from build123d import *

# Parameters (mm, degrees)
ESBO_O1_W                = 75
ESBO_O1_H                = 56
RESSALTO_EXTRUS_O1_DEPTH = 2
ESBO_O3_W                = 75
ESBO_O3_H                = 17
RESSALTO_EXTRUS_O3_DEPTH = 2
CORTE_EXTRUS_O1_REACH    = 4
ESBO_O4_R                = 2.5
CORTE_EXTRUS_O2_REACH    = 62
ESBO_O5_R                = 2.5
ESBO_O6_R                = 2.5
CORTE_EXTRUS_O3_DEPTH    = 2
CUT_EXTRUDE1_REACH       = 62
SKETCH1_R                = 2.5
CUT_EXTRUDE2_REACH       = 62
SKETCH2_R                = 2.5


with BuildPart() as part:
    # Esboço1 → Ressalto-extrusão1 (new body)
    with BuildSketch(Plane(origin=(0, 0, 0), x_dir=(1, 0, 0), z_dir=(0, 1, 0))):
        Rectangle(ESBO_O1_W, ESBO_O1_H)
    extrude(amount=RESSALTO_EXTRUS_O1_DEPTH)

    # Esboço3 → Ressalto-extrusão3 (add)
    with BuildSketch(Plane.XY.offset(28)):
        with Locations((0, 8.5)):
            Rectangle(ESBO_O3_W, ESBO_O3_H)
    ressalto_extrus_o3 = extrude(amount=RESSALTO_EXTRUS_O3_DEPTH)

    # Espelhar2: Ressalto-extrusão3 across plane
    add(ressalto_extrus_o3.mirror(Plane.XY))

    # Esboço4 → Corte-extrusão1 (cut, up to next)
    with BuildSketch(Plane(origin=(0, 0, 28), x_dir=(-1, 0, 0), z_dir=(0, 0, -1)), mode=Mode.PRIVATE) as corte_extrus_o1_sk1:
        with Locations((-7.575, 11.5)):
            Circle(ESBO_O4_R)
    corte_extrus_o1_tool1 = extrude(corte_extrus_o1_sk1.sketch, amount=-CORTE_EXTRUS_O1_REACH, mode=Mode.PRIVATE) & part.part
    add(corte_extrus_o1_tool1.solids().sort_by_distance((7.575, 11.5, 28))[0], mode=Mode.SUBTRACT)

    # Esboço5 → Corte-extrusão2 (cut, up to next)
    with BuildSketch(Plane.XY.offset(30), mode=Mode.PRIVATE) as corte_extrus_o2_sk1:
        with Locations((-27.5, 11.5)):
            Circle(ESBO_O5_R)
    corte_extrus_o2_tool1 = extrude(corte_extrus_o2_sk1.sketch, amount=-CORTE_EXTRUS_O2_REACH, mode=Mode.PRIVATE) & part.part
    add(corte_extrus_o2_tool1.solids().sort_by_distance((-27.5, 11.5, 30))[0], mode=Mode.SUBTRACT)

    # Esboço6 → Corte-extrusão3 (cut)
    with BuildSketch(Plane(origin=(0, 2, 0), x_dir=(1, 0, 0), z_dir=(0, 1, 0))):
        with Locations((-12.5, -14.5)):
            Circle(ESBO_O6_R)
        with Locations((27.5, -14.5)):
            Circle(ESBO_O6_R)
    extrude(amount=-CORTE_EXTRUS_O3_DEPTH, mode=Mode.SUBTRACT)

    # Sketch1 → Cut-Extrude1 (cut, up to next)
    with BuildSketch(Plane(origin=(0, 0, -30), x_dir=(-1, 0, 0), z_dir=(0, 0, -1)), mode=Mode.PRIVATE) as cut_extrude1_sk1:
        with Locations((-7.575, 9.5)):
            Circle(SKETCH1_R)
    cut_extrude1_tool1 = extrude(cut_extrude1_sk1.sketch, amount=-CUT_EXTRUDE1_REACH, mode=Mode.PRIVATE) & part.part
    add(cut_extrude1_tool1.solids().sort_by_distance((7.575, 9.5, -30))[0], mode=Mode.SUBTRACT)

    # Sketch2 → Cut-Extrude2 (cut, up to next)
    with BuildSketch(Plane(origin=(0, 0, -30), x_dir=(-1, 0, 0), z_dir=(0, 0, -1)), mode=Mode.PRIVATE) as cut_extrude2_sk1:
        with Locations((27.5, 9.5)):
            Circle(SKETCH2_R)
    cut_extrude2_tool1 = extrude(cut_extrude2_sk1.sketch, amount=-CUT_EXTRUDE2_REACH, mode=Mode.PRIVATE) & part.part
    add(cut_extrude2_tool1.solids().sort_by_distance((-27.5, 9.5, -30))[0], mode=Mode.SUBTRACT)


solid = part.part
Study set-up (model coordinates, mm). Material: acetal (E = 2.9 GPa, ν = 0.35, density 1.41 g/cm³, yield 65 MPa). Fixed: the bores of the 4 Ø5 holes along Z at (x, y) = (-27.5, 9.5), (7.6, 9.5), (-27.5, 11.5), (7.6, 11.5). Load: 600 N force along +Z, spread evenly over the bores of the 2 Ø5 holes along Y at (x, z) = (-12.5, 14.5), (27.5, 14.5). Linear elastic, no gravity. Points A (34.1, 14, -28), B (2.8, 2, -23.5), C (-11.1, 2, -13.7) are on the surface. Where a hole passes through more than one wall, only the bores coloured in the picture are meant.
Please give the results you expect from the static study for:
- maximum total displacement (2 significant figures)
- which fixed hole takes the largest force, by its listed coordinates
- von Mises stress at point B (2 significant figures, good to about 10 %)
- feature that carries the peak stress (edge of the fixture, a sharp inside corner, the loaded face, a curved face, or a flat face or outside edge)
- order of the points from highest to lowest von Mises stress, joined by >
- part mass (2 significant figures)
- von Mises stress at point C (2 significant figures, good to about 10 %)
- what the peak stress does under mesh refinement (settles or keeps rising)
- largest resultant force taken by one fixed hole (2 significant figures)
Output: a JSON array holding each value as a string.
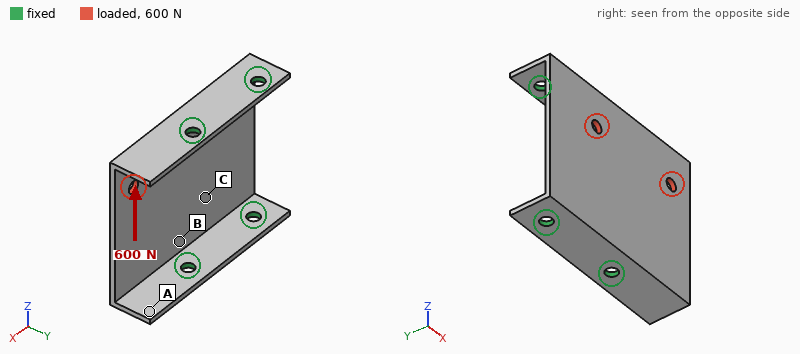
["0.60 mm", "(7.6, 9.5)", "19 MPa", "edge of the fixture", "B > C > A", "19 g", "9.4 MPa", "keeps rising", "220 N"]
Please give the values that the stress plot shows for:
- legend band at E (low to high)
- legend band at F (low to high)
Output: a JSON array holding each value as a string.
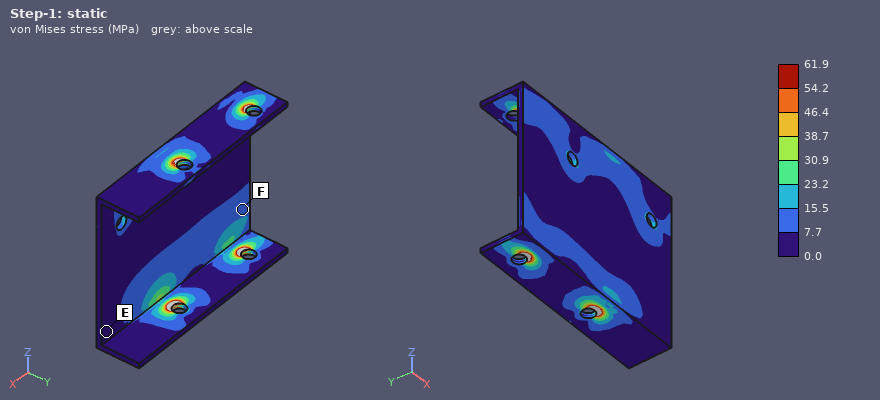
["0.0 to 7.7 MPa", "7.7 to 15.5 MPa"]
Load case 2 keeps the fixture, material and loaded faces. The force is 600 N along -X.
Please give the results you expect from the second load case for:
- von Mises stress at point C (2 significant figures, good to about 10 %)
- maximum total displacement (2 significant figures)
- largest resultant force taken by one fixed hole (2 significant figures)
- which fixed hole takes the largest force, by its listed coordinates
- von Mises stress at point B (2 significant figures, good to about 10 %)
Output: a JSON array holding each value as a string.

["2.5 MPa", "0.27 mm", "260 N", "(7.6, 11.5)", "2.8 MPa"]
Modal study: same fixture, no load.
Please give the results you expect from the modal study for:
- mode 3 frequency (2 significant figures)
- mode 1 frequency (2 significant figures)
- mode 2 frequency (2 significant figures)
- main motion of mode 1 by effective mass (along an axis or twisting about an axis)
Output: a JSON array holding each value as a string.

["1300 Hz", "690 Hz", "850 Hz", "along Y"]
